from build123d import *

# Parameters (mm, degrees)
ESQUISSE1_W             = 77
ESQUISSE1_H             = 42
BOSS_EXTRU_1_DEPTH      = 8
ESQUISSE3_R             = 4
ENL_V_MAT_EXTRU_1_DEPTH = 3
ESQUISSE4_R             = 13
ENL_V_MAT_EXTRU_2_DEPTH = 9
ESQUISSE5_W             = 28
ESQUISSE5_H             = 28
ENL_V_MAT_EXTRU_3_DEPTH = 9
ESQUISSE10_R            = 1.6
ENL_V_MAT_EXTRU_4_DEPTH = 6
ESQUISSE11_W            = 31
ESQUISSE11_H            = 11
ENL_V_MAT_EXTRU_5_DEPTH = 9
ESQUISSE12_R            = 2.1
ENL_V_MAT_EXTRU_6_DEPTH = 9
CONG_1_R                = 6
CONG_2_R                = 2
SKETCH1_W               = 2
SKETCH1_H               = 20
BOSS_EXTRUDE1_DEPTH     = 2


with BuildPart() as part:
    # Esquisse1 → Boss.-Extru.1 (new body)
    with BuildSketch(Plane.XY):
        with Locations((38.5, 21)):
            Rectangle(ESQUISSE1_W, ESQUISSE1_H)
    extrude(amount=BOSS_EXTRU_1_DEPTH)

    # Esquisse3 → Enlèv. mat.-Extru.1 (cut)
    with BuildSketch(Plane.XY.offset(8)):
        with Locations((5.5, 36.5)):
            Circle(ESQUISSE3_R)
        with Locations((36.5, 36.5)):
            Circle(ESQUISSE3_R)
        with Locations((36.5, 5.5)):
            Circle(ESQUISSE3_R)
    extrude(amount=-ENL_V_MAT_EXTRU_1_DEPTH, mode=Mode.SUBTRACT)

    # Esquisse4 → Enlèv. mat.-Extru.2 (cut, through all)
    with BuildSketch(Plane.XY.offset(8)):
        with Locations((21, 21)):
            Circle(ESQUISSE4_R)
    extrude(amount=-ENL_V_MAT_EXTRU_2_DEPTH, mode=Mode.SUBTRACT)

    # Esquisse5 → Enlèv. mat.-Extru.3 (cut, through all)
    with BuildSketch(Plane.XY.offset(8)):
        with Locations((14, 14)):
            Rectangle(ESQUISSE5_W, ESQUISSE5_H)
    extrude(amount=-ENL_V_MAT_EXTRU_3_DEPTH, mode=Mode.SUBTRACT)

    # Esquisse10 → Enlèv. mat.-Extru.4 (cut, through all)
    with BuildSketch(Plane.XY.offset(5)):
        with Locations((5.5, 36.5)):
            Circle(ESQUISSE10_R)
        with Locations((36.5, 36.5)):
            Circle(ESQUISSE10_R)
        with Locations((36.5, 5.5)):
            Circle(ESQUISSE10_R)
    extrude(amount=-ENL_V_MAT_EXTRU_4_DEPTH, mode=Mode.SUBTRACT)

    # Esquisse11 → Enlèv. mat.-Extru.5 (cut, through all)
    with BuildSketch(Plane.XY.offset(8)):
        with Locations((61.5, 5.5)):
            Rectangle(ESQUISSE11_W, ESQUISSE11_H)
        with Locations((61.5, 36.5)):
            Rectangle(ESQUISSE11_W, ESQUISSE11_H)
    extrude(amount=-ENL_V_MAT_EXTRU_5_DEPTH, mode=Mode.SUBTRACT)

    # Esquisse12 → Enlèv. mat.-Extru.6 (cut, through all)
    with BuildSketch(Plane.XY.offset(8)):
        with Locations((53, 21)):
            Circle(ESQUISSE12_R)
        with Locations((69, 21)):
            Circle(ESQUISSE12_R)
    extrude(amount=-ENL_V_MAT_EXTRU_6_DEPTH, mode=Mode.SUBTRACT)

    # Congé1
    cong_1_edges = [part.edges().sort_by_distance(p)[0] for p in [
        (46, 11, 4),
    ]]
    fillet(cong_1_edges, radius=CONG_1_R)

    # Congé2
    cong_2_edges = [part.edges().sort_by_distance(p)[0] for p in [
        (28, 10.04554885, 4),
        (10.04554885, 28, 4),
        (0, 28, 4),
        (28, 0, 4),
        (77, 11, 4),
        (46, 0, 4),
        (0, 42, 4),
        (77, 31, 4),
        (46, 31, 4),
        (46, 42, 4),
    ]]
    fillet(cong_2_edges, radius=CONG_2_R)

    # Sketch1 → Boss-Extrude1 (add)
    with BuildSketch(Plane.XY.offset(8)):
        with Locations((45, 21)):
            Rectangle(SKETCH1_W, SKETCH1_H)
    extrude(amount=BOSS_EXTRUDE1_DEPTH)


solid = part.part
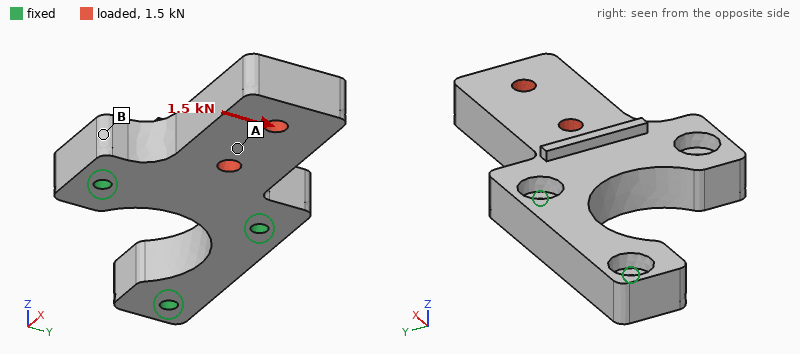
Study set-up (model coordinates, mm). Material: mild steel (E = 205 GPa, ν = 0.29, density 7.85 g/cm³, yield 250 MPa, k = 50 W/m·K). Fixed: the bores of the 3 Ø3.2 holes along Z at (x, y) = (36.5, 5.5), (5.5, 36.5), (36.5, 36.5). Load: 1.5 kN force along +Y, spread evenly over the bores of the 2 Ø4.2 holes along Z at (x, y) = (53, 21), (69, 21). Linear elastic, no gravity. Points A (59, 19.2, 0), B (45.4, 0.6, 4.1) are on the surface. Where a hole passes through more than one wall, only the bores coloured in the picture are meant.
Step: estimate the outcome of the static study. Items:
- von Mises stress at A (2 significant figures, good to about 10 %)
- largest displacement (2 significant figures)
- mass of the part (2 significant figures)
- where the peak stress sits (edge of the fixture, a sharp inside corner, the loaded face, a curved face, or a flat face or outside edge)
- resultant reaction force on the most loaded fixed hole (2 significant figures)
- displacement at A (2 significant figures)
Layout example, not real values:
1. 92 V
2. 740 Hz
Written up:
1. 17 MPa
2. 12 µm
3. 94 g
4. a curved face
5. 1.4 kN
6. 5.5 µm
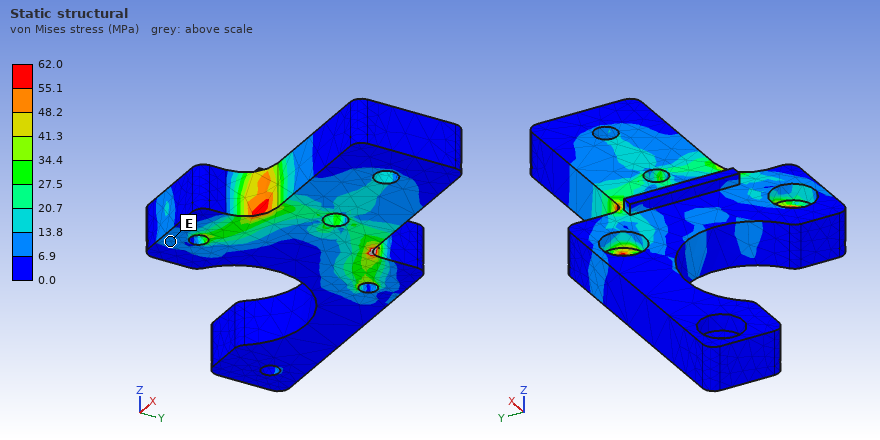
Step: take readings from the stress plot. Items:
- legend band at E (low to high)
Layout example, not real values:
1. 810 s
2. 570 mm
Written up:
1. 6.9 to 13.8 MPa
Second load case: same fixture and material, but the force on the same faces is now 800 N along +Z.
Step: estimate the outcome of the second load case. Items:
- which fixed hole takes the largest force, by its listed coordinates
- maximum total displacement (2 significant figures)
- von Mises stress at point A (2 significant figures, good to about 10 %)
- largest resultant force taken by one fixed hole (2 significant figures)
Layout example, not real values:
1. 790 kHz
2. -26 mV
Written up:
1. (36.5, 36.5)
2. 75 µm
3. 22 MPa
4. 630 N
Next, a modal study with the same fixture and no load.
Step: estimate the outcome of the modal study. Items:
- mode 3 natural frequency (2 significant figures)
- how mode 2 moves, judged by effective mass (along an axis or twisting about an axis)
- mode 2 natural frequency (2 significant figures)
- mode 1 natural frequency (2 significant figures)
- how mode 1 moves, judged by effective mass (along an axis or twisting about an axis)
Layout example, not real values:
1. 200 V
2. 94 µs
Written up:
1. 14 kHz
2. along Y
3. 11 kHz
4. 3200 Hz
5. along Z
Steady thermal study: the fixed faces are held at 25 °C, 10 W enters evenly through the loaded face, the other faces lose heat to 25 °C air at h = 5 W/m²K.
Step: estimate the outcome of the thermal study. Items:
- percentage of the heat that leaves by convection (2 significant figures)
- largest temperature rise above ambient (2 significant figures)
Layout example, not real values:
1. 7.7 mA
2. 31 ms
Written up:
1. 3.2 %
2. 35 K
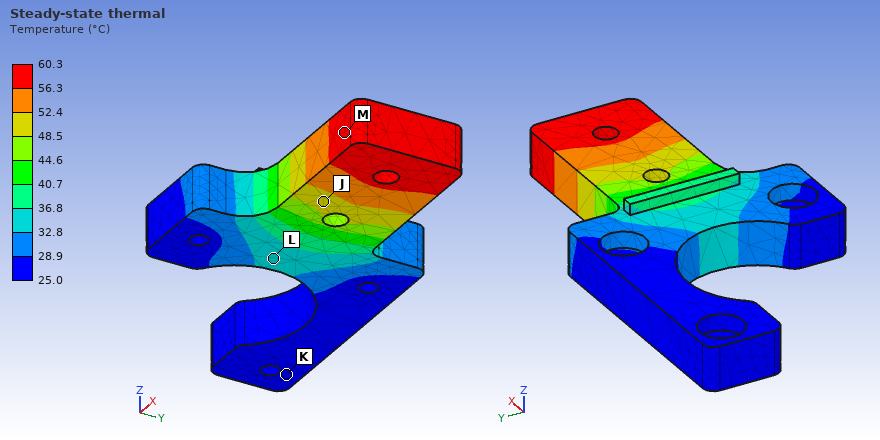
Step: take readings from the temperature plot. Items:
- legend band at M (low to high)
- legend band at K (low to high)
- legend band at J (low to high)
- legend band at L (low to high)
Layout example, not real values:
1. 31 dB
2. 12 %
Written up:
1. 56.3 to 60.3 °C
2. 25.0 to 28.9 °C
3. 48.5 to 52.4 °C
4. 32.8 to 36.8 °C
